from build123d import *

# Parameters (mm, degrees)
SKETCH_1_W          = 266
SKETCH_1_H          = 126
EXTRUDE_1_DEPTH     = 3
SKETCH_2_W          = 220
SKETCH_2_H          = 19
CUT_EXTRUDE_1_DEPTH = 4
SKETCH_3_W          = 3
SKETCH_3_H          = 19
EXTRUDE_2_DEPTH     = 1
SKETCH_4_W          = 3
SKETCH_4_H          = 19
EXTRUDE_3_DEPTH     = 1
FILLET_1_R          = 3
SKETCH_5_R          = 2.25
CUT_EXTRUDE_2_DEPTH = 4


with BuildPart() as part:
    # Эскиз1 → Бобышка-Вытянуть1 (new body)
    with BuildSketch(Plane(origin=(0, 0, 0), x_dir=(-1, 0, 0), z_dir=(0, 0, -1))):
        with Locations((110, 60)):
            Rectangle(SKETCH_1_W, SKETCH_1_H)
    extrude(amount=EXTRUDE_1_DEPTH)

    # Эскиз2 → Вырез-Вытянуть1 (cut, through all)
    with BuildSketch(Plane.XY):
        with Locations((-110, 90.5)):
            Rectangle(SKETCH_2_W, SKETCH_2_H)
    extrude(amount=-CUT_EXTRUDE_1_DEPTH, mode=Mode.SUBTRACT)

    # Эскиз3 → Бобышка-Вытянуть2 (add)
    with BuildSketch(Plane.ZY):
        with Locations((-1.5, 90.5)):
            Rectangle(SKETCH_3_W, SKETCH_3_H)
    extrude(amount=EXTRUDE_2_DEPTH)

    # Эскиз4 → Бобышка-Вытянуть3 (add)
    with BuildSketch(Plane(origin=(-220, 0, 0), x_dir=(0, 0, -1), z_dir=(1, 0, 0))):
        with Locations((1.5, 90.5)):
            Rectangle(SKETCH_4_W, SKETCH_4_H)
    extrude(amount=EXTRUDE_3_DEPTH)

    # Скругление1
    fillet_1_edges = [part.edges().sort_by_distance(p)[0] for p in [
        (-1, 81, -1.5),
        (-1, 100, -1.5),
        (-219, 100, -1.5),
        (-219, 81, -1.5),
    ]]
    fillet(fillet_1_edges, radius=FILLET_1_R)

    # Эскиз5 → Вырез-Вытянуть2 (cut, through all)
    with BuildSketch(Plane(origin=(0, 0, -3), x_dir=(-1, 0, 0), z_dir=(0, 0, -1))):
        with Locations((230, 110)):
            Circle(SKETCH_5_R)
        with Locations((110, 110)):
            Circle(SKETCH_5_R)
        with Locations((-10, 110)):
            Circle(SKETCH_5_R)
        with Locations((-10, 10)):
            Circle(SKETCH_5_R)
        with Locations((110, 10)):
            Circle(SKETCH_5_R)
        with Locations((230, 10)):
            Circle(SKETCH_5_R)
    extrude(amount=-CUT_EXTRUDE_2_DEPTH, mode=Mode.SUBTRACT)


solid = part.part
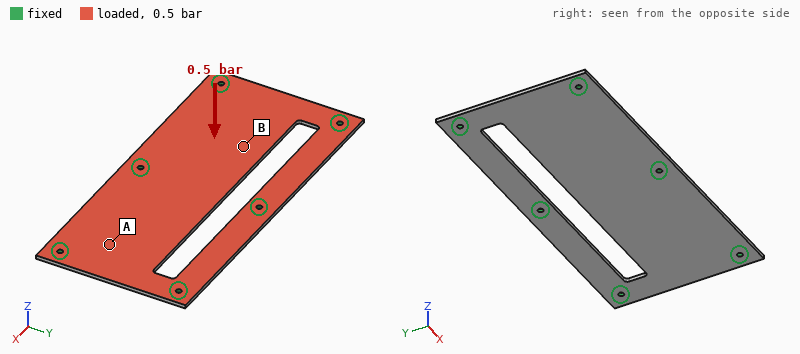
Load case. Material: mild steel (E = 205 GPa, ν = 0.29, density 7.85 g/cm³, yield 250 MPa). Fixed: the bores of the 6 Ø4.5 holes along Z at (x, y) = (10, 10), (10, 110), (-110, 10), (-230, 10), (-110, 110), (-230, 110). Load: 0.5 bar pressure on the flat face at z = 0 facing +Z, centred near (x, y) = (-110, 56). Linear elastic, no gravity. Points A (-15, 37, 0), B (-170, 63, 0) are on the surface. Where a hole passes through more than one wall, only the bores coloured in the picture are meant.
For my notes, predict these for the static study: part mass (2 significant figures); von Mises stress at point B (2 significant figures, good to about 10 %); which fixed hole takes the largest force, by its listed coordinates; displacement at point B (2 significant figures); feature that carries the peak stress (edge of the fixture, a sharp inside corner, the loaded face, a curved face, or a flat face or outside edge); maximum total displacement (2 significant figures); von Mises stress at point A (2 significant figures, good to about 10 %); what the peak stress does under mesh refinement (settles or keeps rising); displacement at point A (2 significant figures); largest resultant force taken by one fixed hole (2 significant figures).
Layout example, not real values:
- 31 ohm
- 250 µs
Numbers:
- 690 g
- 33 MPa
- (-110, 10)
- 0.24 mm
- edge of the fixture
- 0.39 mm
- 12 MPa
- keeps rising
- 0.091 mm
- 500 N
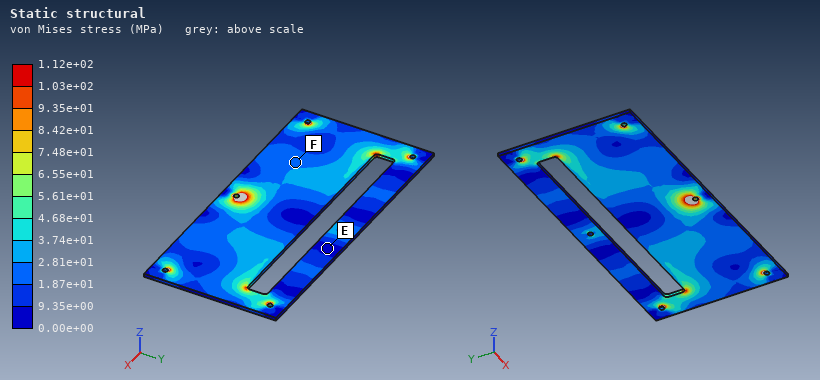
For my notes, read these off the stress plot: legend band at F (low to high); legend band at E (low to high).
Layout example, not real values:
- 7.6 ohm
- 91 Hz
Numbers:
- 1.87e+01 to 2.81e+01 MPa
- 0.00e+00 to 9.35e+00 MPa
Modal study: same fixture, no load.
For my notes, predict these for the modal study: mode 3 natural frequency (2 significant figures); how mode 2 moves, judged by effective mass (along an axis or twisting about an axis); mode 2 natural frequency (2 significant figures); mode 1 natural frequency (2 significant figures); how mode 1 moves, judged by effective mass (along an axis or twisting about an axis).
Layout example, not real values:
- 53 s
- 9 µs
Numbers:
- 1100 Hz
- twisting about Y
- 720 Hz
- 500 Hz
- along Z
